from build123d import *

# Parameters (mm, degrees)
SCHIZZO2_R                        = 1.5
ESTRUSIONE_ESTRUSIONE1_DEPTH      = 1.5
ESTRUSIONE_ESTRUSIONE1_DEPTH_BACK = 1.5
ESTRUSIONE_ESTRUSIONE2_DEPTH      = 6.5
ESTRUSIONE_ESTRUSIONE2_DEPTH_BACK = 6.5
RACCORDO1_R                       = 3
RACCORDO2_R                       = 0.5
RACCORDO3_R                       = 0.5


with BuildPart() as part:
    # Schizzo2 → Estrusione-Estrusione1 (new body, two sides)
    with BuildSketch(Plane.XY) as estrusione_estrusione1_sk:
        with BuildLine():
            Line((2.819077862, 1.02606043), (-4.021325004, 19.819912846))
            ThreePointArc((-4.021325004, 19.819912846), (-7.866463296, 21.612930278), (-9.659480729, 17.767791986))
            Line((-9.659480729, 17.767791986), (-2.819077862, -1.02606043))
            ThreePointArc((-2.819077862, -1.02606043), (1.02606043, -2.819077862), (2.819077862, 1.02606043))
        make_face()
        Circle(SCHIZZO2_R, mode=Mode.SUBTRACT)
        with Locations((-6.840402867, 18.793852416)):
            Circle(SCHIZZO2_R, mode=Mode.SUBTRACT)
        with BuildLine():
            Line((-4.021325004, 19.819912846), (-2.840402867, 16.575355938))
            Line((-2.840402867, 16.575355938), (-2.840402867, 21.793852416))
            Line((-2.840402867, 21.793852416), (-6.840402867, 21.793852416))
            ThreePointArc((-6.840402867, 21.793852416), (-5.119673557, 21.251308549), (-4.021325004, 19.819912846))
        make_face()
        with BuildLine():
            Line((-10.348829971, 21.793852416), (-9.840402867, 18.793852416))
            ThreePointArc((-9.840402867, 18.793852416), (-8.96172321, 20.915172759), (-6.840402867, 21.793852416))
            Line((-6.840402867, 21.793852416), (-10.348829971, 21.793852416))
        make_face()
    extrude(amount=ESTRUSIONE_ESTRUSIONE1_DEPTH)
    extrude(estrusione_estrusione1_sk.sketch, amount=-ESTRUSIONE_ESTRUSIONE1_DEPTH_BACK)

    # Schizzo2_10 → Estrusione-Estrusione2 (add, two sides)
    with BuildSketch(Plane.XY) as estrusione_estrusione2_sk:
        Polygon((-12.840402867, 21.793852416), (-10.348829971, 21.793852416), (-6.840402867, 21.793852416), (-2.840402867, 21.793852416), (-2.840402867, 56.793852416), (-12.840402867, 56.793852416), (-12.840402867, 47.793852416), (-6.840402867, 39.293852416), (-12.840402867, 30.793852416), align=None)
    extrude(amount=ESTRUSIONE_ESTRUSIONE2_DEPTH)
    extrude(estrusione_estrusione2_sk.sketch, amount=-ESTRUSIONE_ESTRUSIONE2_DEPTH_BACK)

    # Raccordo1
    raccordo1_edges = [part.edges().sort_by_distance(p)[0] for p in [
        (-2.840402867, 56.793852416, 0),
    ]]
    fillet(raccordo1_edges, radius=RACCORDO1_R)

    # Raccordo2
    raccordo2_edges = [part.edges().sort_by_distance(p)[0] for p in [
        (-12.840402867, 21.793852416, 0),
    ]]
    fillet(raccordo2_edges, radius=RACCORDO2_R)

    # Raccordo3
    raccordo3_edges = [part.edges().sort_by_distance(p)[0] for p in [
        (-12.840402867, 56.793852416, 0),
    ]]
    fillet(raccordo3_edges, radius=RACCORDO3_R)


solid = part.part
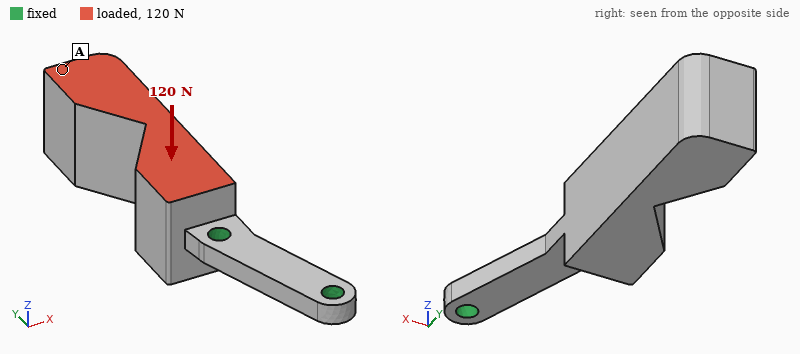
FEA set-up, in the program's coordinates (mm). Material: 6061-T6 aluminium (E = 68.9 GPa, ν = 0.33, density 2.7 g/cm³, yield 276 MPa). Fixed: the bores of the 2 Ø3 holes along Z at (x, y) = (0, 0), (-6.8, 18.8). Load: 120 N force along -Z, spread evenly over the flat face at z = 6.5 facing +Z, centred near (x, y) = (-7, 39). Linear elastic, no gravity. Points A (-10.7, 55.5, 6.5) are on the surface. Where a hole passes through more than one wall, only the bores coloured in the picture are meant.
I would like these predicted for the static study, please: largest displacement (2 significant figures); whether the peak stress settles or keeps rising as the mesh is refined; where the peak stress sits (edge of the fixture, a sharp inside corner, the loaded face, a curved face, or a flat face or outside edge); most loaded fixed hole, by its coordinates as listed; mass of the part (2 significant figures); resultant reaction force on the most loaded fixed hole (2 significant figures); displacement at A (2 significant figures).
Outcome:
0.22 mm
keeps rising
edge of the fixture
(-6.8, 18.8)
12 g
120 N
0.21 mm
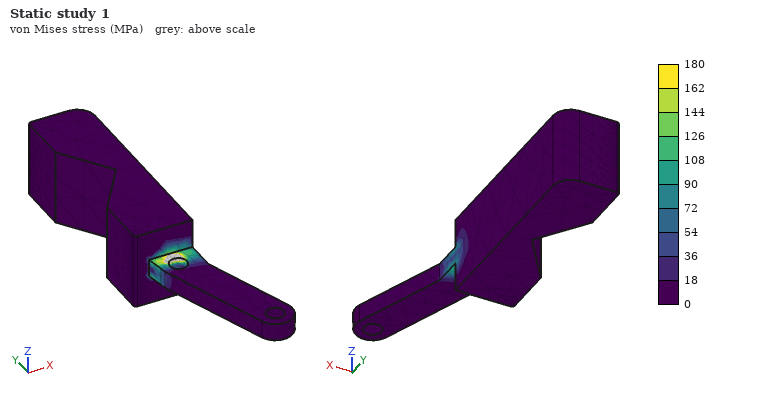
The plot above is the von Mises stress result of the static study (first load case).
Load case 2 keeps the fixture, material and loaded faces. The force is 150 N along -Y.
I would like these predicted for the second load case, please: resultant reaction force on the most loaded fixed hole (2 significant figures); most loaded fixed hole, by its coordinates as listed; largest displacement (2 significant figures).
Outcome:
150 N
(-6.8, 18.8)
0.10 mm
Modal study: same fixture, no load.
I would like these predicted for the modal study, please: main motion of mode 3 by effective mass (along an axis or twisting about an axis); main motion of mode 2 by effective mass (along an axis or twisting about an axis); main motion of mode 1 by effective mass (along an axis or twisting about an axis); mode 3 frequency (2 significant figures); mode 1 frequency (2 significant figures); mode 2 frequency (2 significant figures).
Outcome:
twisting about Y
along X
along Z
7600 Hz
1400 Hz
2100 Hz
